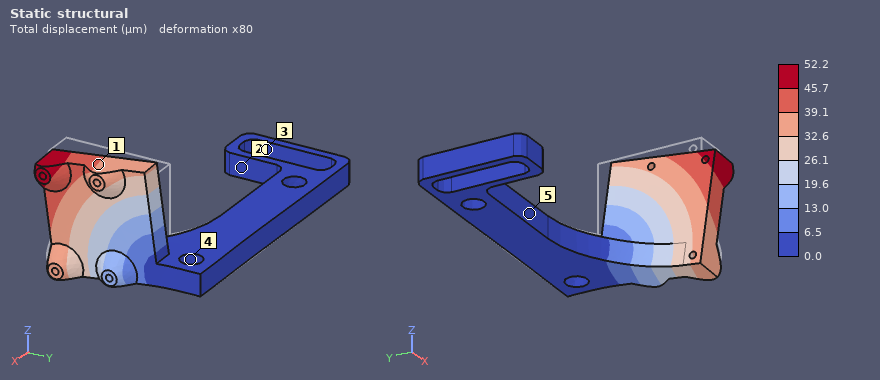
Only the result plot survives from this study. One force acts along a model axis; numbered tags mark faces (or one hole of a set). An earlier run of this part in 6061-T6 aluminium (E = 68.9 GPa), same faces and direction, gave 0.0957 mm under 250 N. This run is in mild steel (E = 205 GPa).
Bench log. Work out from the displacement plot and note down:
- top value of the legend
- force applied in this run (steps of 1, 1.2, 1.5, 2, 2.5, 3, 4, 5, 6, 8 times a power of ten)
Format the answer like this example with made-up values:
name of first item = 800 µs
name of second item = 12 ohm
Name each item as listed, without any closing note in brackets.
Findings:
top value of the legend = 52.2 µm
force applied in this run = 400 N
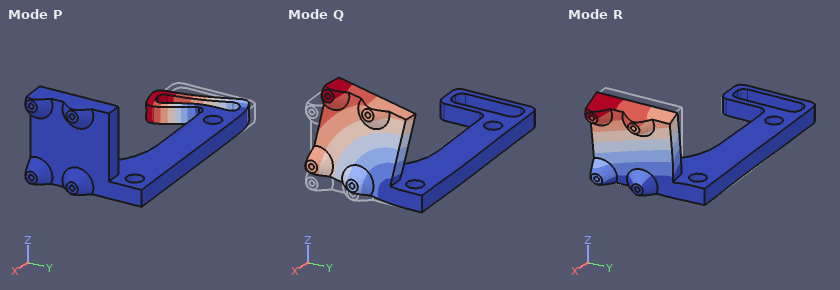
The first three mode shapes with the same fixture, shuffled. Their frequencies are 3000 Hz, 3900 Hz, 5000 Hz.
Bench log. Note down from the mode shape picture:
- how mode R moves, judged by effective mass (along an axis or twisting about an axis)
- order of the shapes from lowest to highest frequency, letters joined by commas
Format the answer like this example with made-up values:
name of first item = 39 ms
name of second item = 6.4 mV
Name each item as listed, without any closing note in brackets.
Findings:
how mode R moves, judged by effective mass = along X
order of the shapes from lowest to highest frequency, letters joined by commas = Q, R, P
